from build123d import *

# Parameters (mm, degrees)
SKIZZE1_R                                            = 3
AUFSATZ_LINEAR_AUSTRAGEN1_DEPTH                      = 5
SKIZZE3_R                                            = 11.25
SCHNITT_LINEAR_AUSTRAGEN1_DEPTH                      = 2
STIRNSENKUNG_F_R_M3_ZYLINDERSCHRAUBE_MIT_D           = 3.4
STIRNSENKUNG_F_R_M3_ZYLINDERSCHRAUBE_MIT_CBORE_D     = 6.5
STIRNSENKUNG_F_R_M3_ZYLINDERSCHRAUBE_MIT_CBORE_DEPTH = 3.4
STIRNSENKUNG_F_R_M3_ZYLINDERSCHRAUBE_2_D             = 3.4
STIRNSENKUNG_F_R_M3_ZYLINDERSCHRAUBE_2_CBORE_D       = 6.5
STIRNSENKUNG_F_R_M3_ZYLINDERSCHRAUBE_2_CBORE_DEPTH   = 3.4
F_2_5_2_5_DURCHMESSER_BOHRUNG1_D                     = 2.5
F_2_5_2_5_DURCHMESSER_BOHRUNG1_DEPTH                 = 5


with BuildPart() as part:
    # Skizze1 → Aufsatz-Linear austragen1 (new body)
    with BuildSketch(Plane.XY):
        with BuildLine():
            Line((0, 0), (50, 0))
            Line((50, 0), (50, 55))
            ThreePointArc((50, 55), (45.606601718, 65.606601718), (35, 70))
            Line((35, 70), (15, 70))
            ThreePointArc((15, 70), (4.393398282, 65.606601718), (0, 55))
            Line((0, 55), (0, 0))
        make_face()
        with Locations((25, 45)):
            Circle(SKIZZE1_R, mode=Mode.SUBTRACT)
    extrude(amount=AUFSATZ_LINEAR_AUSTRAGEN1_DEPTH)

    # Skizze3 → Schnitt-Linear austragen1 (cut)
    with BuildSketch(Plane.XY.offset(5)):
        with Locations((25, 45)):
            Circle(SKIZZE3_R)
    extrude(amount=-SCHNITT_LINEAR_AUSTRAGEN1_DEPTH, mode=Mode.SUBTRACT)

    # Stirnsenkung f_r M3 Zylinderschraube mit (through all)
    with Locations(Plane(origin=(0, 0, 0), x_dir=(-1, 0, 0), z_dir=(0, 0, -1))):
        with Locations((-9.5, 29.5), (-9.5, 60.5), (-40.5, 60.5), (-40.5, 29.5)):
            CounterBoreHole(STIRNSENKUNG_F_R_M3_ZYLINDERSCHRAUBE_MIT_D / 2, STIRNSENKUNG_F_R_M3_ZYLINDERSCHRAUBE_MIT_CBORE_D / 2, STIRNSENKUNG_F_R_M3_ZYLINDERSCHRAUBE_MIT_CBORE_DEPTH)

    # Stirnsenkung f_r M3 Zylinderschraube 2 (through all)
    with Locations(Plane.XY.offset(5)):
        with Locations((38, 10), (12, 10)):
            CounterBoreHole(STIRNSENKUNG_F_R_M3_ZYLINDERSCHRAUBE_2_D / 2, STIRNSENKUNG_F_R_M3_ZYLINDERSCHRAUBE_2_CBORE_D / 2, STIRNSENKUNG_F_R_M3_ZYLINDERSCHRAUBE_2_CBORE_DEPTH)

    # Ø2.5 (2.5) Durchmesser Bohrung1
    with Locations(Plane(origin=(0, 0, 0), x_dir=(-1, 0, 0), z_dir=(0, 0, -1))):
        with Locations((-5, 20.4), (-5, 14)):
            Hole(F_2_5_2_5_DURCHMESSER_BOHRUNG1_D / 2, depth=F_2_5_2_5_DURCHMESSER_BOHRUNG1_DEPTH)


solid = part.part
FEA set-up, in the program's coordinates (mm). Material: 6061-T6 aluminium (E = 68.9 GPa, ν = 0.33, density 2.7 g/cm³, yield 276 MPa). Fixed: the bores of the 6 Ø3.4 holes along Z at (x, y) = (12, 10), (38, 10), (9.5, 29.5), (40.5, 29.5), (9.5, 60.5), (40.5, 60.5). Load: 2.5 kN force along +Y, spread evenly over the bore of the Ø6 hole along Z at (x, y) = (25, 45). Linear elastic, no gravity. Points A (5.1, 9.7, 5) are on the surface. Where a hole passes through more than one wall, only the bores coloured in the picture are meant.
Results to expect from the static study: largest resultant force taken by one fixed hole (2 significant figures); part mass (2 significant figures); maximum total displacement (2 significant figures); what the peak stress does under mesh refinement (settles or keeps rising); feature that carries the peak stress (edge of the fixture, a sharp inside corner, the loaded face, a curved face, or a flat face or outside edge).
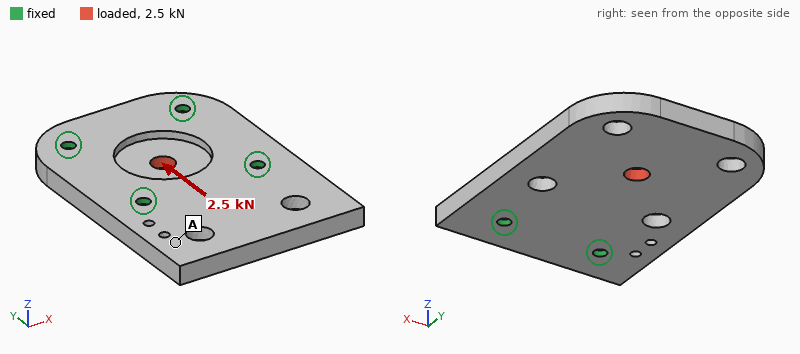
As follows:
510 N
41 g
8.9 µm
keeps rising
edge of the fixture
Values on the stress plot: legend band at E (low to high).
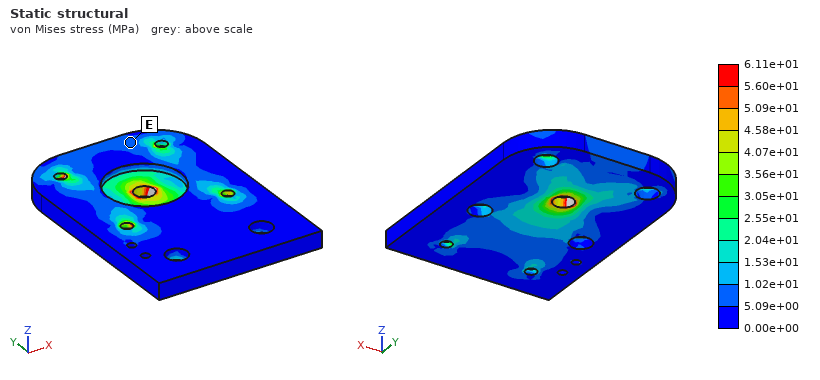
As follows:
5.09e+00 to 1.02e+01 MPa
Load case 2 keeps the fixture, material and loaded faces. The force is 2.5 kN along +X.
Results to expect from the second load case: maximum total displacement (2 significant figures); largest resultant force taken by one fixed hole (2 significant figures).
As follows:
9.5 µm
640 N
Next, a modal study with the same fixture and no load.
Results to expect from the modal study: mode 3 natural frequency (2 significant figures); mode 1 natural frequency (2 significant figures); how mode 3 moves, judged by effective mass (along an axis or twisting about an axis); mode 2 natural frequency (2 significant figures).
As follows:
16 kHz
14 kHz
twisting about Y
14 kHz
